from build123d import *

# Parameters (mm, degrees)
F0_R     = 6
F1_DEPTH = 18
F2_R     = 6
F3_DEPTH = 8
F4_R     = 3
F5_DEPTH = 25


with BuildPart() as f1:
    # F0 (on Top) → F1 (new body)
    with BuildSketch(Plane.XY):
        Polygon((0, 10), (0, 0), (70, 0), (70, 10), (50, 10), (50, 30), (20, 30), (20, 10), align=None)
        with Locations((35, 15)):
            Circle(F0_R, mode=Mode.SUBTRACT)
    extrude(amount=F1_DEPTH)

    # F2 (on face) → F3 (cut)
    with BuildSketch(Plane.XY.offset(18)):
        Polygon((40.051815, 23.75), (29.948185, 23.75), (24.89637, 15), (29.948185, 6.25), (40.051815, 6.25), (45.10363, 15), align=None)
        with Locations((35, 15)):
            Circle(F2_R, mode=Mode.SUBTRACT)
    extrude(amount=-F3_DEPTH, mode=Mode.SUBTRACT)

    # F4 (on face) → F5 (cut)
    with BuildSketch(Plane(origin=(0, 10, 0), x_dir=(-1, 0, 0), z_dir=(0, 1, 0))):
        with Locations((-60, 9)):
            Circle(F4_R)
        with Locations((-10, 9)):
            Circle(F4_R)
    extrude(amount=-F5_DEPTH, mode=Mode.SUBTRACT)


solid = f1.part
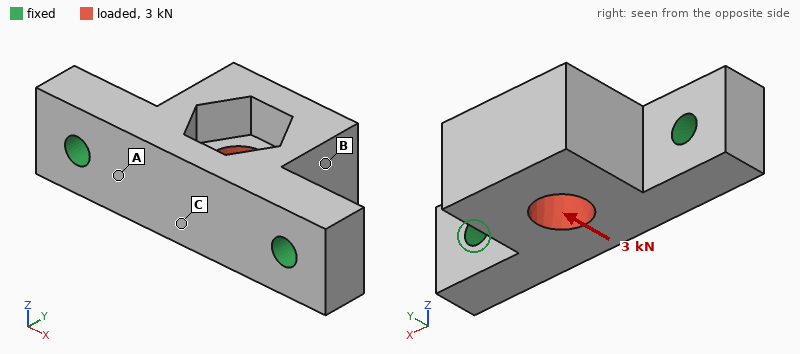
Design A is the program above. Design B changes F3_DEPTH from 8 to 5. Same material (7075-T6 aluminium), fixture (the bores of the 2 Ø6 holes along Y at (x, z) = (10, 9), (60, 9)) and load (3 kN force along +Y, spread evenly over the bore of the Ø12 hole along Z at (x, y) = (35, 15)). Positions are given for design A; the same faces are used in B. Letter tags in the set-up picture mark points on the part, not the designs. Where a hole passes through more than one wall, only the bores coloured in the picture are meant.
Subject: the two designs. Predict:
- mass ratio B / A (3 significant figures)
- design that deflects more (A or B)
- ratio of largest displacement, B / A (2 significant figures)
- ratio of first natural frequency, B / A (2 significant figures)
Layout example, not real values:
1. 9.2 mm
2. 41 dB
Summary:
1. 1.02
2. A
3. 0.72
4. 0.99
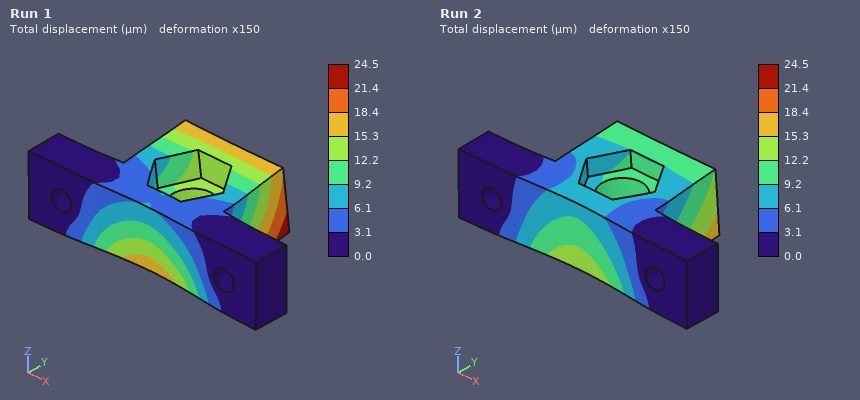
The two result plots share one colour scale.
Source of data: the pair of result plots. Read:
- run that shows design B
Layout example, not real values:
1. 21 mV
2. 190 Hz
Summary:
1. Run 2
